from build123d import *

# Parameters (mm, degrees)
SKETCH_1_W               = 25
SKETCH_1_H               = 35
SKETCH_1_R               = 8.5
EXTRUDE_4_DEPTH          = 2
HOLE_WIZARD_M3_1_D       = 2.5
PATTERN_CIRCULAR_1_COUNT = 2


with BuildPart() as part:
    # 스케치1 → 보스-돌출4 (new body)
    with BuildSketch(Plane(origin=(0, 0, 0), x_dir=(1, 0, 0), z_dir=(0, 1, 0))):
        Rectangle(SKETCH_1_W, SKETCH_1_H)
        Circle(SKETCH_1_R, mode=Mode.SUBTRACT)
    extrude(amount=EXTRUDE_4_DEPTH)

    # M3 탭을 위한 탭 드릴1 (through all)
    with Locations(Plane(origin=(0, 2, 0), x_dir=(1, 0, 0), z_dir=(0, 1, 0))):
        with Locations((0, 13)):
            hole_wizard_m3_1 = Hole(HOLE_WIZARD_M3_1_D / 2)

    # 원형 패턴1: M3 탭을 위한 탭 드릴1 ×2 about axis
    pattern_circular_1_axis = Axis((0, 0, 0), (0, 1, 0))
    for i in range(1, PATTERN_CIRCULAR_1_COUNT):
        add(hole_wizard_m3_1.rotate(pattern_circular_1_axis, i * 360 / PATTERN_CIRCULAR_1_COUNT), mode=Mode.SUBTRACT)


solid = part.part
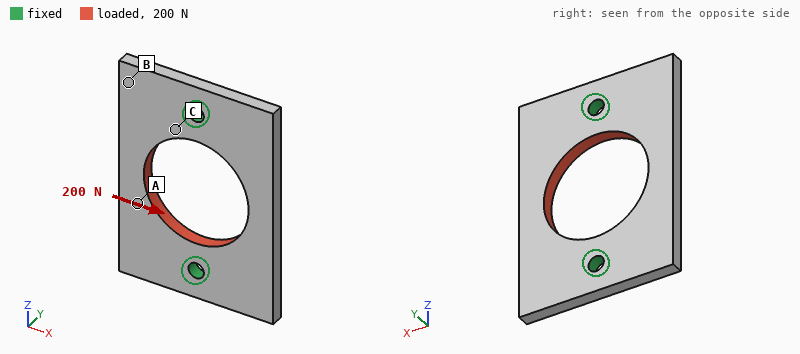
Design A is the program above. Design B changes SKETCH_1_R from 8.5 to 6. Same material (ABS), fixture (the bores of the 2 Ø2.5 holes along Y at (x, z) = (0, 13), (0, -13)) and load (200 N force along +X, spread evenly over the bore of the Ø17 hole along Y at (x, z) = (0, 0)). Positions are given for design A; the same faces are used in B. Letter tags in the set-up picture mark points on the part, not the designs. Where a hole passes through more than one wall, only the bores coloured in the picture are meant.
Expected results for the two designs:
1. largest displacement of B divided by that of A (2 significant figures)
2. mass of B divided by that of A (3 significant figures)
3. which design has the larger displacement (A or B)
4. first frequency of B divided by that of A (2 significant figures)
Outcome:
0.83
1.18
A
0.99
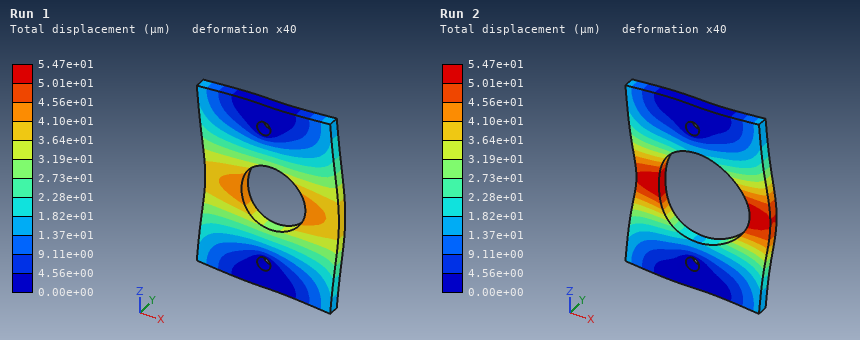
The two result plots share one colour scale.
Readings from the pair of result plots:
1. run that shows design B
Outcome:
Run 1
